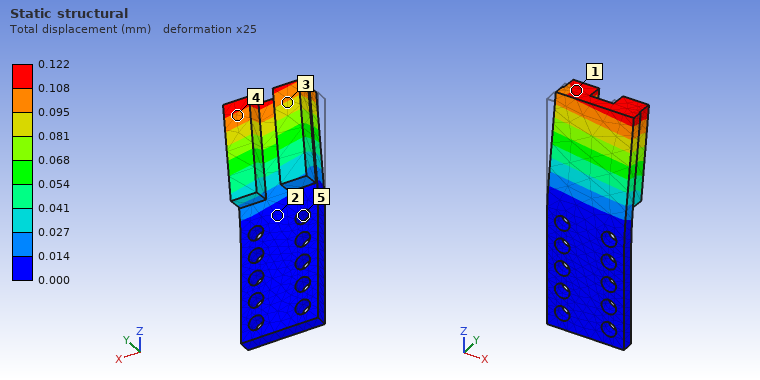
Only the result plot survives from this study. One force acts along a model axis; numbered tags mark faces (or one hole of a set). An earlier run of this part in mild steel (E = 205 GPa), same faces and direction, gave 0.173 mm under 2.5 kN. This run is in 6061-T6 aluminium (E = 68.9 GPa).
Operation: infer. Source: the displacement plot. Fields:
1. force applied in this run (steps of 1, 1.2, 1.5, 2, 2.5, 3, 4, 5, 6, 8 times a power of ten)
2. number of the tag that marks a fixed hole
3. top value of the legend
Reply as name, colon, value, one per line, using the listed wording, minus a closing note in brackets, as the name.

force applied in this run: 600 N
number of the tag that marks a fixed hole: 5
top value of the legend: 0.122 mm
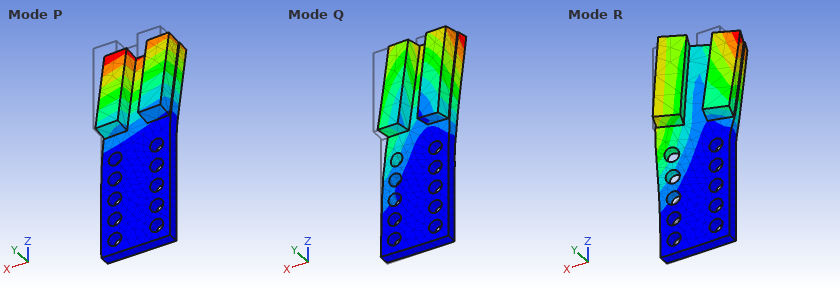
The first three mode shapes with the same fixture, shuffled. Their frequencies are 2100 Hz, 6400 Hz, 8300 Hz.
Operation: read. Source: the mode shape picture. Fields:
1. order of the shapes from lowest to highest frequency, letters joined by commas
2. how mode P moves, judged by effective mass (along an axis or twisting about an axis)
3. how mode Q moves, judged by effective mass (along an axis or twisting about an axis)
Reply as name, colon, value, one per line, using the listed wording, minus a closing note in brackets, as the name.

order of the shapes from lowest to highest frequency, letters joined by commas: P, R, Q
how mode P moves, judged by effective mass: along Y
how mode Q moves, judged by effective mass: along X
